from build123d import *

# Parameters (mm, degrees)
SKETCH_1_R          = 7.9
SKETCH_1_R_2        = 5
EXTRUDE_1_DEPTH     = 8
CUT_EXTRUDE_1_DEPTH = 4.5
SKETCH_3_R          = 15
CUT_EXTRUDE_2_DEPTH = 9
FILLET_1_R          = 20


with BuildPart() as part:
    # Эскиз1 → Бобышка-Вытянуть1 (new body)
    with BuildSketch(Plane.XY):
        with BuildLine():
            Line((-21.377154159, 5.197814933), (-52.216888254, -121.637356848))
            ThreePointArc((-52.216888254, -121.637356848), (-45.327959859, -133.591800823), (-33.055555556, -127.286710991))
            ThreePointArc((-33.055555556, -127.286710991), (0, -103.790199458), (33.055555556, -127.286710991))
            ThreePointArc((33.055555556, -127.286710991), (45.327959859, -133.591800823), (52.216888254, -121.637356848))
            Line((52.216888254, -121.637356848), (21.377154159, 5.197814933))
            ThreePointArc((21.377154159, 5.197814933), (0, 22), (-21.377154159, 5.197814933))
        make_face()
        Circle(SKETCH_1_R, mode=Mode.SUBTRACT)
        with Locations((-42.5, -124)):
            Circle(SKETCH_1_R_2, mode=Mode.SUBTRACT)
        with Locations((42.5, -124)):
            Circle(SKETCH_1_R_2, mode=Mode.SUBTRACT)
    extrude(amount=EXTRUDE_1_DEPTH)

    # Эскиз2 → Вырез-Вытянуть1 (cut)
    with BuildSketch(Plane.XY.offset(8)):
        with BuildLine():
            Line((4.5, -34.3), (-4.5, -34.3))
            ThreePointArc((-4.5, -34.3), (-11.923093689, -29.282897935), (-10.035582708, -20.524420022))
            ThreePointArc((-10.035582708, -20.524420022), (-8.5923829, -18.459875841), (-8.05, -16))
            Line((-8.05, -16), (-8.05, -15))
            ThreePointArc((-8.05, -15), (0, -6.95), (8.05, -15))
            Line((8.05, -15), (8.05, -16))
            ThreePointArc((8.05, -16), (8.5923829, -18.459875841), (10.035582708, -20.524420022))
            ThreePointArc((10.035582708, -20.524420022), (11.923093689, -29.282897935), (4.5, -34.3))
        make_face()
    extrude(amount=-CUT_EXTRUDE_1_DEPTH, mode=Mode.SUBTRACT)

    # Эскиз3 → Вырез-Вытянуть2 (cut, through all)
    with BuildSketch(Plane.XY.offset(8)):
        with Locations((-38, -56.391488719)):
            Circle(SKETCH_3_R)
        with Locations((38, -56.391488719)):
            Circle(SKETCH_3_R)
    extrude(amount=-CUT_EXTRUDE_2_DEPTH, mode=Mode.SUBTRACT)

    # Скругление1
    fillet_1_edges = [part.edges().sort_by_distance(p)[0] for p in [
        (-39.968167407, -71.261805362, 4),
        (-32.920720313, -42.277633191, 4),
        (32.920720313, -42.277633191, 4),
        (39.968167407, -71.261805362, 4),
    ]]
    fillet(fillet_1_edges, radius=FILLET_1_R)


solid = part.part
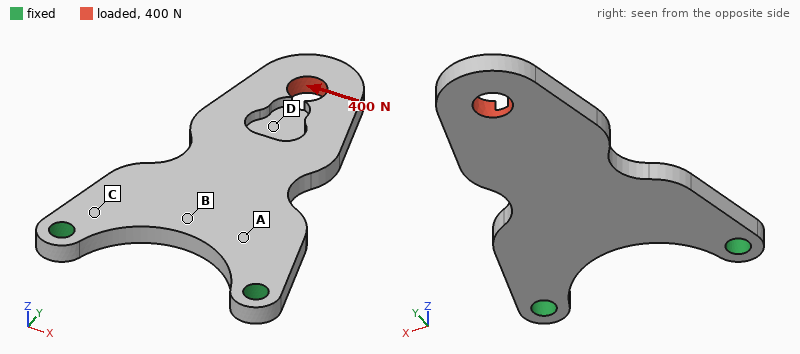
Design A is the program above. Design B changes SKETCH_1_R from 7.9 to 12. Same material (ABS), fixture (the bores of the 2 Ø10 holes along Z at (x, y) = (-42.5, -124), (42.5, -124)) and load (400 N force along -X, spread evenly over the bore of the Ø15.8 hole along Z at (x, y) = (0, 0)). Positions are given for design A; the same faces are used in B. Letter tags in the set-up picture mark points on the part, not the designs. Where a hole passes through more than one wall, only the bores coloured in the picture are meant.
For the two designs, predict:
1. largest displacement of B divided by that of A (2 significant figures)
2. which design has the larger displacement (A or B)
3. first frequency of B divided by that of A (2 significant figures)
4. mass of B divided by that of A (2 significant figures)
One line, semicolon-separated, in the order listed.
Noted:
1.1; B; 1.1; 0.97
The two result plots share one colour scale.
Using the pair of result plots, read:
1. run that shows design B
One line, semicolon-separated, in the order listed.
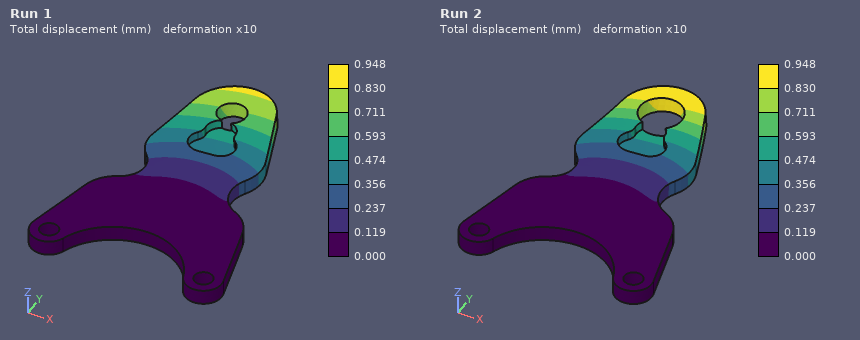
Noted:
Run 2
